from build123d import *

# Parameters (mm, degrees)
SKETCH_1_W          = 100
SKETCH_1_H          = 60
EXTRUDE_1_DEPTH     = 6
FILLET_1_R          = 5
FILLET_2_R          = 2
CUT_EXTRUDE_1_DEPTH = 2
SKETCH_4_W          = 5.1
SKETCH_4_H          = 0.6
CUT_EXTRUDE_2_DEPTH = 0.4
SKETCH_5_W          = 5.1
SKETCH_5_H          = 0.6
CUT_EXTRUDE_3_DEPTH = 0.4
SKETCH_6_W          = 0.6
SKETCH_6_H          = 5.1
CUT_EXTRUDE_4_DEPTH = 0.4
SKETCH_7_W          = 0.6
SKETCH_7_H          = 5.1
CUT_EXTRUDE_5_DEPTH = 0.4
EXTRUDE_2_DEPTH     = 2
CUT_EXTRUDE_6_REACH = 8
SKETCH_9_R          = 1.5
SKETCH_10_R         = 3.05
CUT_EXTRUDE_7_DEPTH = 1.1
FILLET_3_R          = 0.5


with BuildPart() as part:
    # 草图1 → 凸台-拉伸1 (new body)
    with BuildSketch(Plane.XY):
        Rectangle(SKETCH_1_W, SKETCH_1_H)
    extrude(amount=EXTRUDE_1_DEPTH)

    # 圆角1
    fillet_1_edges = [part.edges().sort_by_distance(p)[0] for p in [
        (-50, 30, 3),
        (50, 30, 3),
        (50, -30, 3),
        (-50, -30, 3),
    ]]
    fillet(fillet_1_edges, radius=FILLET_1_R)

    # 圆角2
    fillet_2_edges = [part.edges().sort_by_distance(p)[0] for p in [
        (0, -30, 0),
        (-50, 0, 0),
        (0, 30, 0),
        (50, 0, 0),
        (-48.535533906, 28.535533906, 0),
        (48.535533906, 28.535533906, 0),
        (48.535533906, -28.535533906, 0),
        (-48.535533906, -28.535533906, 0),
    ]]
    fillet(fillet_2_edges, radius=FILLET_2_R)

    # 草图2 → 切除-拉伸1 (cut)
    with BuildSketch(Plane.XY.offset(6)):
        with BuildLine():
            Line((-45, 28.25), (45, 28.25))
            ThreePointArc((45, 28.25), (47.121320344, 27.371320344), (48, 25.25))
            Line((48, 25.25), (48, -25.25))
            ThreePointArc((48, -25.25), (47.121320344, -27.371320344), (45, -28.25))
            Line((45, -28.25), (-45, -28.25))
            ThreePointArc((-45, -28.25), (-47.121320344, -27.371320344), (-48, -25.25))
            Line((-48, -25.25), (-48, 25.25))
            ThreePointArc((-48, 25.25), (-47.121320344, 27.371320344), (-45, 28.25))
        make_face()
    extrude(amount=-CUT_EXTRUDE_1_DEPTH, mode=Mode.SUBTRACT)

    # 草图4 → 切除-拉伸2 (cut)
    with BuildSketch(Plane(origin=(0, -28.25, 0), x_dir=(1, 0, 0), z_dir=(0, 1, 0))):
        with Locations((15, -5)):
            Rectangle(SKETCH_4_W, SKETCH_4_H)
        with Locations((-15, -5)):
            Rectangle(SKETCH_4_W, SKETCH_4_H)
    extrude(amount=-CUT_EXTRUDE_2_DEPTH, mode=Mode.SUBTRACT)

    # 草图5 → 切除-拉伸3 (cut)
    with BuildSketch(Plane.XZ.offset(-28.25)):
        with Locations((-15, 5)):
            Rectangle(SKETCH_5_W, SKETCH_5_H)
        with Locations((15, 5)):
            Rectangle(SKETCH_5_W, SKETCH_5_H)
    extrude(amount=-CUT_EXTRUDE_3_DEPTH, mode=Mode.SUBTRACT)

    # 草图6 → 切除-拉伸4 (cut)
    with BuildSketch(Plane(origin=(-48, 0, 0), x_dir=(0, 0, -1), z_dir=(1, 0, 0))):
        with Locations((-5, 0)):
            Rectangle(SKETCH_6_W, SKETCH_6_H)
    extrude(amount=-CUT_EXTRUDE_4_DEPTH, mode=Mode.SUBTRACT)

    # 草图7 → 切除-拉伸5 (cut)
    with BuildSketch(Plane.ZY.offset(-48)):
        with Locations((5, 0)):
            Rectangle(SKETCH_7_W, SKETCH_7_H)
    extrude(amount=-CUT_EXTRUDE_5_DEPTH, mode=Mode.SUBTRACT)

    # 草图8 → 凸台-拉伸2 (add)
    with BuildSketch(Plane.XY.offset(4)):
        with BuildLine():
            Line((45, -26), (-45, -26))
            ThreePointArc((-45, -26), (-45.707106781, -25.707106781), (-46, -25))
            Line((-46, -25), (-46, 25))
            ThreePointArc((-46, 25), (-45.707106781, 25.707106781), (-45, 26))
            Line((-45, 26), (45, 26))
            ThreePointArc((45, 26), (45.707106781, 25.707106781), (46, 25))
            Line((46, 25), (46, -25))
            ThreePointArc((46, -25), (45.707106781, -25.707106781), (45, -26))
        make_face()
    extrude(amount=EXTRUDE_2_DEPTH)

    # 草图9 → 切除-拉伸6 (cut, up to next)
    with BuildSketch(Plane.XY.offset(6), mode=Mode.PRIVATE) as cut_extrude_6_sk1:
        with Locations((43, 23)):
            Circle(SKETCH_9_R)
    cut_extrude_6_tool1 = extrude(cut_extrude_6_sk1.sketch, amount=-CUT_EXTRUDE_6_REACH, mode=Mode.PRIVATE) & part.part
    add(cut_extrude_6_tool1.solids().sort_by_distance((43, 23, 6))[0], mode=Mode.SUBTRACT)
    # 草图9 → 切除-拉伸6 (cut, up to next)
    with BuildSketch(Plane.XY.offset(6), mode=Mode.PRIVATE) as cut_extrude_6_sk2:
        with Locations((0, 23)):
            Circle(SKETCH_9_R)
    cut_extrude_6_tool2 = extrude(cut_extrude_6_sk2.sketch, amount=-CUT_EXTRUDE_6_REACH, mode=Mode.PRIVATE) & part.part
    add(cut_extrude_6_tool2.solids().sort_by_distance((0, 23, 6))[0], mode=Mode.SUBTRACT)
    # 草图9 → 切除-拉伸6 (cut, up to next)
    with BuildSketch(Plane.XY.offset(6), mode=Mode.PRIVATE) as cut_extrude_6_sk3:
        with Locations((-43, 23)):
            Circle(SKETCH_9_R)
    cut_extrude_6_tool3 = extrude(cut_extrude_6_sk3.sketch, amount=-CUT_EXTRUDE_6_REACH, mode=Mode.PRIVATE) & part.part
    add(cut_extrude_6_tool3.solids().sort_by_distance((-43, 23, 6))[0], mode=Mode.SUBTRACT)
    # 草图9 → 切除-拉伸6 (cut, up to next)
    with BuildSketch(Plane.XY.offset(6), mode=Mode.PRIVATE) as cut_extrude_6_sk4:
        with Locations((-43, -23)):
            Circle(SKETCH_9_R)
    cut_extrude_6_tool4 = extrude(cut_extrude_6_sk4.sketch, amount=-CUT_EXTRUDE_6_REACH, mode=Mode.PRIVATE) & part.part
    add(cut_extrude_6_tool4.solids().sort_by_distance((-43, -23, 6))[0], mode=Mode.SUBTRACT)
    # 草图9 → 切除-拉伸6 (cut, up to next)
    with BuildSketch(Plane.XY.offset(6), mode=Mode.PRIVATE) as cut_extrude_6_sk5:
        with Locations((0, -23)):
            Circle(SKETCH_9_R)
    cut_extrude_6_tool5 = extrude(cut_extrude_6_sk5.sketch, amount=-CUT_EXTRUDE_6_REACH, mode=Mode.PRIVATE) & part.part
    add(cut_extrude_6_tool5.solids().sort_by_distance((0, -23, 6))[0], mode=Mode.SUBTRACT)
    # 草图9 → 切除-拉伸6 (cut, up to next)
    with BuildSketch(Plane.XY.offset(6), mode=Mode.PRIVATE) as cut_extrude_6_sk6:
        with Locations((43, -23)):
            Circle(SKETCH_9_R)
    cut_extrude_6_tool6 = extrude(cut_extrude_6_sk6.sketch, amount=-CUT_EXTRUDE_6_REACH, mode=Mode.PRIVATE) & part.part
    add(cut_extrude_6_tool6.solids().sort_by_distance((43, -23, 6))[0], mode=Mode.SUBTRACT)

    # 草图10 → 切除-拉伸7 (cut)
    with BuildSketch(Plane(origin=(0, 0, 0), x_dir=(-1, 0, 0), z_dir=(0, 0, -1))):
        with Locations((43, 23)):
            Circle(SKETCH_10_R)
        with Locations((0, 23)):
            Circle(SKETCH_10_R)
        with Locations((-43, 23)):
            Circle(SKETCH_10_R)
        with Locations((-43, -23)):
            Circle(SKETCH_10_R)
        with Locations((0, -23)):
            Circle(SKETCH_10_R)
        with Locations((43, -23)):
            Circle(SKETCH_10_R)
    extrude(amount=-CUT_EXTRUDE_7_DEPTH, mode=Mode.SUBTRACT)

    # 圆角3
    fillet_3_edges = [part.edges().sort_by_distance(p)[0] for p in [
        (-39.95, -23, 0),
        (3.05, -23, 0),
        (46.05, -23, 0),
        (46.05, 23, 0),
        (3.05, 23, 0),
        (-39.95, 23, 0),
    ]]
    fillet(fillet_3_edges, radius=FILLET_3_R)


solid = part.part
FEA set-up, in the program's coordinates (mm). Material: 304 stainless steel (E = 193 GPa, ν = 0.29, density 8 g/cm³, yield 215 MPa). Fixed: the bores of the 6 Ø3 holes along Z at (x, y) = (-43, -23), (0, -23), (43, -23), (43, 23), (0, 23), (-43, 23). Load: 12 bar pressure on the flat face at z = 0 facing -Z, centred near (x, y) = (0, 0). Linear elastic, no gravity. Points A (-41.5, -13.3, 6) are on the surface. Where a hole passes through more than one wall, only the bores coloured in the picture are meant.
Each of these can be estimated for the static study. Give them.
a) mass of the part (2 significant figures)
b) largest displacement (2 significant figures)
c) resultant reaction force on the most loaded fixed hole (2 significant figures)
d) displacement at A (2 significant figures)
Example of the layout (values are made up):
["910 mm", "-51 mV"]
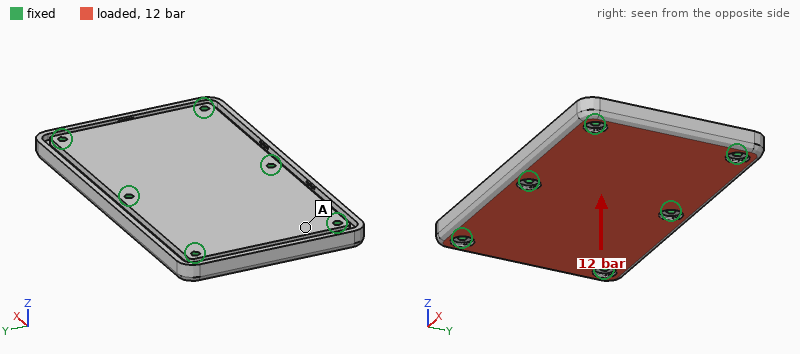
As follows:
["270 g", "13 µm", "1.5 kN", "5.3 µm"]
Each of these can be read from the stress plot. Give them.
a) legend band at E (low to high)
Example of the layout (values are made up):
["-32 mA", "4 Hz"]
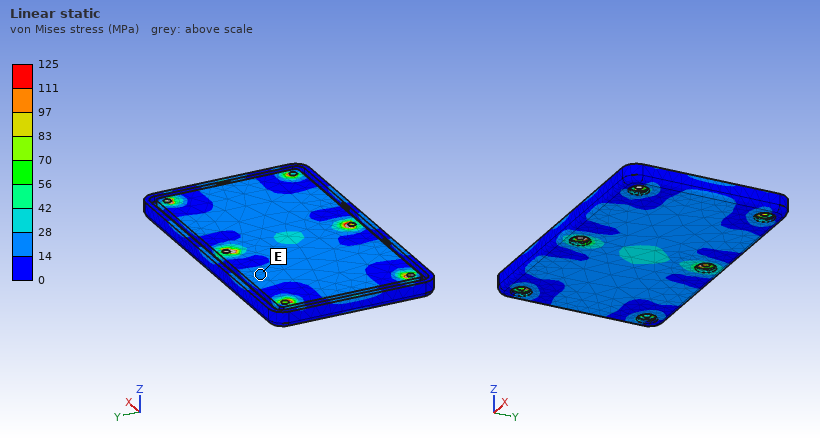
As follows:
["14 to 28 MPa"]
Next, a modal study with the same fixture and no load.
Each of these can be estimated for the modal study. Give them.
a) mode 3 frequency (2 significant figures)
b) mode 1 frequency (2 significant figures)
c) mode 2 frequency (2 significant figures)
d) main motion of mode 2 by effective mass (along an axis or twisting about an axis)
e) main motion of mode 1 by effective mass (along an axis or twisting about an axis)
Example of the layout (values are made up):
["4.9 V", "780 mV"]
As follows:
["13 kHz", "8100 Hz", "8800 Hz", "twisting about Y", "along Z"]
